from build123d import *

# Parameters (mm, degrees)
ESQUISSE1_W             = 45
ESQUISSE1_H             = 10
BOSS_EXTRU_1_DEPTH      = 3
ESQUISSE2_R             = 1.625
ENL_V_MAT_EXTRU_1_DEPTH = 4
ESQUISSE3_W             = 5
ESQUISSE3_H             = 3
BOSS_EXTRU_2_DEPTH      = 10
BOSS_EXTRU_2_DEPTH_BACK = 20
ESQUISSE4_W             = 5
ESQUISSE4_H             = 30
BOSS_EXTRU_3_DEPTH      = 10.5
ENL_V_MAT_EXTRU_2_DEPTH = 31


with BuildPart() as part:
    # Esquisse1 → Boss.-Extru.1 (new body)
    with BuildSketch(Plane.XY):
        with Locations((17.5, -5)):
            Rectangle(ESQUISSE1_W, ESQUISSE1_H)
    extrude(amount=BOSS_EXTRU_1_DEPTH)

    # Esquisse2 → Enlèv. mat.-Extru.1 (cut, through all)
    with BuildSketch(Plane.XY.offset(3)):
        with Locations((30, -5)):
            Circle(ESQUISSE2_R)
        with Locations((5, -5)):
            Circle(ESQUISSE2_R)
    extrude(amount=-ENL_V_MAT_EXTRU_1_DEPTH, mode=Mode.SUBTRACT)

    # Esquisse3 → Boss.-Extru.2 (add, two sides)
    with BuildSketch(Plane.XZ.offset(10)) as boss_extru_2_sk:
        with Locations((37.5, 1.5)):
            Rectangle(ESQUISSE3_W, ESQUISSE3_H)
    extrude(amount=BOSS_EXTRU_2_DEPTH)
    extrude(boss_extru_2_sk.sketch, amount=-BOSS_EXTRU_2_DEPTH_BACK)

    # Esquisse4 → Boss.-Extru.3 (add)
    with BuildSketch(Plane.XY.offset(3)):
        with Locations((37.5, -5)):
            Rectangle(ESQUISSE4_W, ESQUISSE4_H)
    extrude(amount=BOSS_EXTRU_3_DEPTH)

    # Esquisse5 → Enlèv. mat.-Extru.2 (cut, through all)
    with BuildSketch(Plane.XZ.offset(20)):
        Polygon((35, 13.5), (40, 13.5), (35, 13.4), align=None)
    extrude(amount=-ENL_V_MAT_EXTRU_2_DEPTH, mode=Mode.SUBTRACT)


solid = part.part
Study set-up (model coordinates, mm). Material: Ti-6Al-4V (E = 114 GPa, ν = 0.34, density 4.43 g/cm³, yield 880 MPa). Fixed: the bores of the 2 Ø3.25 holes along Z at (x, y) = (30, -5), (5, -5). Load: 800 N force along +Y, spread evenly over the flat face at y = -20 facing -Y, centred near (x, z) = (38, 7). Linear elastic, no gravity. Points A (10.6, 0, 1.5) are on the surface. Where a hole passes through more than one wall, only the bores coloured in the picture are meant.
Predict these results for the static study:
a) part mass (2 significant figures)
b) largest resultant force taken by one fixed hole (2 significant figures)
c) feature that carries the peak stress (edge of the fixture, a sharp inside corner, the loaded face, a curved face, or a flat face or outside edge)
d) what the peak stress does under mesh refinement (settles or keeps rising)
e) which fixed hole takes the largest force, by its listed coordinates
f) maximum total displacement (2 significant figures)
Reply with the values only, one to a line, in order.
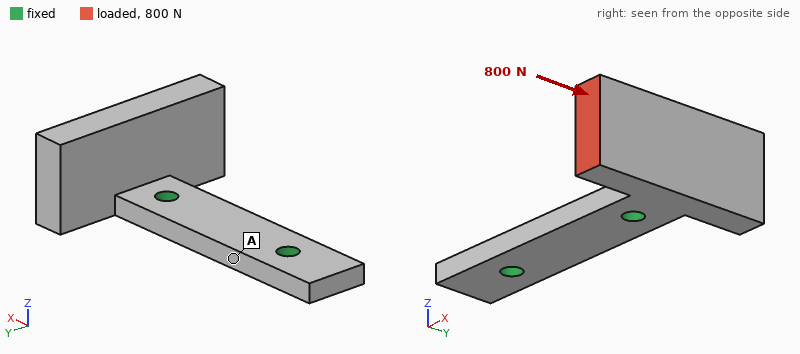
14 g
900 N
edge of the fixture
keeps rising
(30, -5)
0.11 mm
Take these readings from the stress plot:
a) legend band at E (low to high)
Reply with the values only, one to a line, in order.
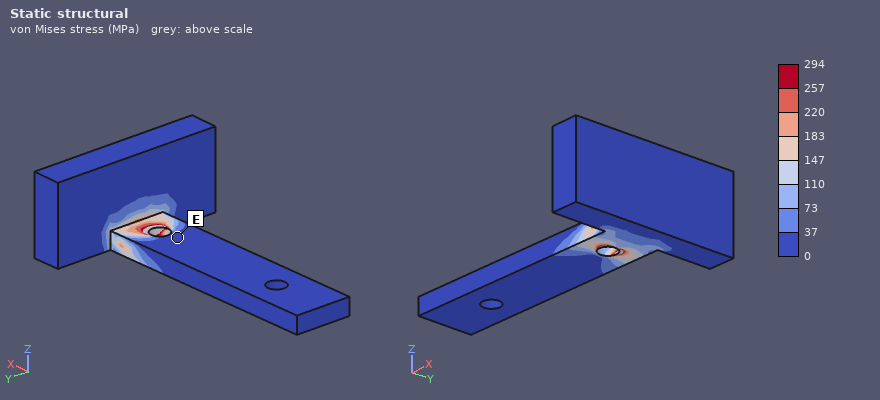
0 to 37 MPa
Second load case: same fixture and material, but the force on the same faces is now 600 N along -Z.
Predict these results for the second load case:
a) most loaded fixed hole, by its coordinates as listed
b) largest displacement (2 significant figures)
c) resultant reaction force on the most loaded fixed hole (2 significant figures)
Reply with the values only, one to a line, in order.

(30, -5)
0.26 mm
610 N
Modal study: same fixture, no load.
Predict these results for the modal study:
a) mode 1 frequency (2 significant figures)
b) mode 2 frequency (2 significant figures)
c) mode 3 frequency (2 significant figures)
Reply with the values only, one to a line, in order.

4400 Hz
4600 Hz
7800 Hz
